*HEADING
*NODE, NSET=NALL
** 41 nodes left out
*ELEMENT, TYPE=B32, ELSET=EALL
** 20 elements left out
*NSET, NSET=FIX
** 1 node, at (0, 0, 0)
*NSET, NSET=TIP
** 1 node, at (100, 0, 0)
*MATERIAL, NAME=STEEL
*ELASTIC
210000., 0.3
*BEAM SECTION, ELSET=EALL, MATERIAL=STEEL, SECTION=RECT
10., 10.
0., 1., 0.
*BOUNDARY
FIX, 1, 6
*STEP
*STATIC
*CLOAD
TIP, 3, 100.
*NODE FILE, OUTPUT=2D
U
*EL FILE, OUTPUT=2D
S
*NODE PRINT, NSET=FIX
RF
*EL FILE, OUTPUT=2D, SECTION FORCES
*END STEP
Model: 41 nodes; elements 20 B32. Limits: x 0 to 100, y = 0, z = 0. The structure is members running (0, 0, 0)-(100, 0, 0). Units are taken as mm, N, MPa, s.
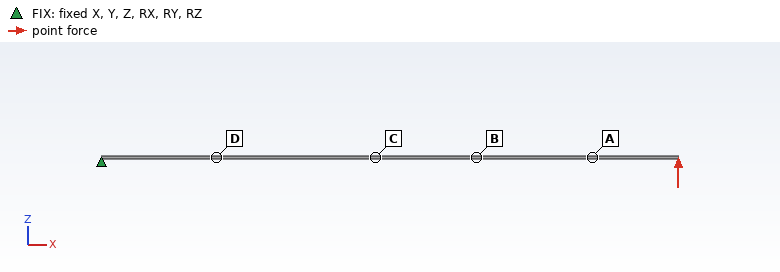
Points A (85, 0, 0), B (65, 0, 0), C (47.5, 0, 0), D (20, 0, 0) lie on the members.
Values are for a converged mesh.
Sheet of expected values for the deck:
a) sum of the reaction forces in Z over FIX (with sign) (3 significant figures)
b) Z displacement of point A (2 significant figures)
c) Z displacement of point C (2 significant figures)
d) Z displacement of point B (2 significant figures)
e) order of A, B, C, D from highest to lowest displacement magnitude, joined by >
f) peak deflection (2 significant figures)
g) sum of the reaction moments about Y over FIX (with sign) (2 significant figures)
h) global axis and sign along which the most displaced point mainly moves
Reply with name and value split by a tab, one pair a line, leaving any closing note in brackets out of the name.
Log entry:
sum of the reaction forces in Z over FIX (with sign)	-100 N
Z displacement of point A	0.15 mm
Z displacement of point C	0.055 mm
Z displacement of point B	0.096 mm
order of A, B, C, D from highest to lowest displacement magnitude, joined by >	A > B > C > D
peak deflection	0.19 mm
sum of the reaction moments about Y over FIX (with sign)	10000 N·mm
global axis and sign along which the most displaced point mainly moves	+Z
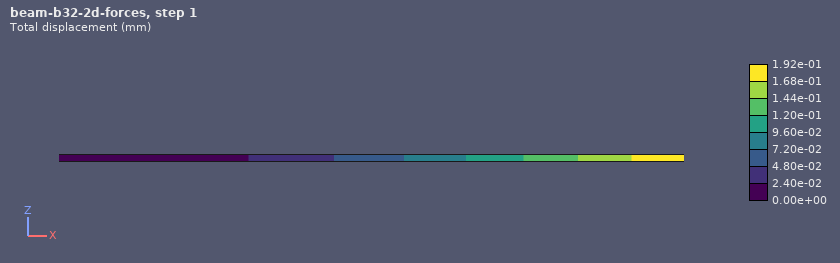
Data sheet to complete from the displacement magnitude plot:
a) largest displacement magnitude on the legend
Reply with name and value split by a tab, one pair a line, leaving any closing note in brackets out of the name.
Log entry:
largest displacement magnitude on the legend	1.92e-01 mm
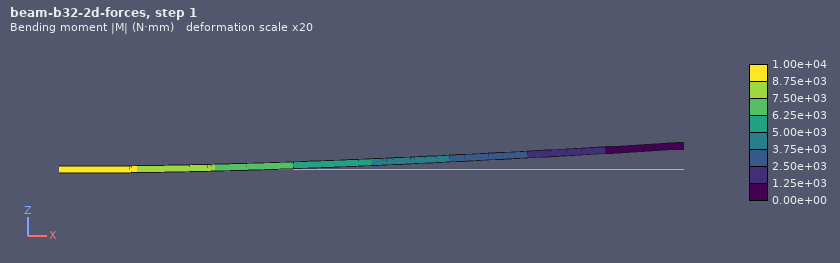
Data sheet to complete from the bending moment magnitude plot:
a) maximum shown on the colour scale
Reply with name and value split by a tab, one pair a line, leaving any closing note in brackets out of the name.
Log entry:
maximum shown on the colour scale	1.00e+04 N·mm
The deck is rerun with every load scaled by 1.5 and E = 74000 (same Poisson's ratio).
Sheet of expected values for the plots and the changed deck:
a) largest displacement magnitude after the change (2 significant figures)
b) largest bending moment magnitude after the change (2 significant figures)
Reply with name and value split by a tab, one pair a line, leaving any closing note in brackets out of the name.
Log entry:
largest displacement magnitude after the change	0.82 mm
largest bending moment magnitude after the change	15000 N·mm
